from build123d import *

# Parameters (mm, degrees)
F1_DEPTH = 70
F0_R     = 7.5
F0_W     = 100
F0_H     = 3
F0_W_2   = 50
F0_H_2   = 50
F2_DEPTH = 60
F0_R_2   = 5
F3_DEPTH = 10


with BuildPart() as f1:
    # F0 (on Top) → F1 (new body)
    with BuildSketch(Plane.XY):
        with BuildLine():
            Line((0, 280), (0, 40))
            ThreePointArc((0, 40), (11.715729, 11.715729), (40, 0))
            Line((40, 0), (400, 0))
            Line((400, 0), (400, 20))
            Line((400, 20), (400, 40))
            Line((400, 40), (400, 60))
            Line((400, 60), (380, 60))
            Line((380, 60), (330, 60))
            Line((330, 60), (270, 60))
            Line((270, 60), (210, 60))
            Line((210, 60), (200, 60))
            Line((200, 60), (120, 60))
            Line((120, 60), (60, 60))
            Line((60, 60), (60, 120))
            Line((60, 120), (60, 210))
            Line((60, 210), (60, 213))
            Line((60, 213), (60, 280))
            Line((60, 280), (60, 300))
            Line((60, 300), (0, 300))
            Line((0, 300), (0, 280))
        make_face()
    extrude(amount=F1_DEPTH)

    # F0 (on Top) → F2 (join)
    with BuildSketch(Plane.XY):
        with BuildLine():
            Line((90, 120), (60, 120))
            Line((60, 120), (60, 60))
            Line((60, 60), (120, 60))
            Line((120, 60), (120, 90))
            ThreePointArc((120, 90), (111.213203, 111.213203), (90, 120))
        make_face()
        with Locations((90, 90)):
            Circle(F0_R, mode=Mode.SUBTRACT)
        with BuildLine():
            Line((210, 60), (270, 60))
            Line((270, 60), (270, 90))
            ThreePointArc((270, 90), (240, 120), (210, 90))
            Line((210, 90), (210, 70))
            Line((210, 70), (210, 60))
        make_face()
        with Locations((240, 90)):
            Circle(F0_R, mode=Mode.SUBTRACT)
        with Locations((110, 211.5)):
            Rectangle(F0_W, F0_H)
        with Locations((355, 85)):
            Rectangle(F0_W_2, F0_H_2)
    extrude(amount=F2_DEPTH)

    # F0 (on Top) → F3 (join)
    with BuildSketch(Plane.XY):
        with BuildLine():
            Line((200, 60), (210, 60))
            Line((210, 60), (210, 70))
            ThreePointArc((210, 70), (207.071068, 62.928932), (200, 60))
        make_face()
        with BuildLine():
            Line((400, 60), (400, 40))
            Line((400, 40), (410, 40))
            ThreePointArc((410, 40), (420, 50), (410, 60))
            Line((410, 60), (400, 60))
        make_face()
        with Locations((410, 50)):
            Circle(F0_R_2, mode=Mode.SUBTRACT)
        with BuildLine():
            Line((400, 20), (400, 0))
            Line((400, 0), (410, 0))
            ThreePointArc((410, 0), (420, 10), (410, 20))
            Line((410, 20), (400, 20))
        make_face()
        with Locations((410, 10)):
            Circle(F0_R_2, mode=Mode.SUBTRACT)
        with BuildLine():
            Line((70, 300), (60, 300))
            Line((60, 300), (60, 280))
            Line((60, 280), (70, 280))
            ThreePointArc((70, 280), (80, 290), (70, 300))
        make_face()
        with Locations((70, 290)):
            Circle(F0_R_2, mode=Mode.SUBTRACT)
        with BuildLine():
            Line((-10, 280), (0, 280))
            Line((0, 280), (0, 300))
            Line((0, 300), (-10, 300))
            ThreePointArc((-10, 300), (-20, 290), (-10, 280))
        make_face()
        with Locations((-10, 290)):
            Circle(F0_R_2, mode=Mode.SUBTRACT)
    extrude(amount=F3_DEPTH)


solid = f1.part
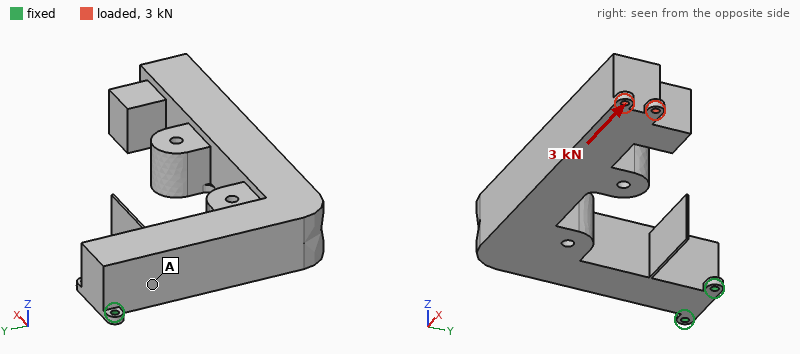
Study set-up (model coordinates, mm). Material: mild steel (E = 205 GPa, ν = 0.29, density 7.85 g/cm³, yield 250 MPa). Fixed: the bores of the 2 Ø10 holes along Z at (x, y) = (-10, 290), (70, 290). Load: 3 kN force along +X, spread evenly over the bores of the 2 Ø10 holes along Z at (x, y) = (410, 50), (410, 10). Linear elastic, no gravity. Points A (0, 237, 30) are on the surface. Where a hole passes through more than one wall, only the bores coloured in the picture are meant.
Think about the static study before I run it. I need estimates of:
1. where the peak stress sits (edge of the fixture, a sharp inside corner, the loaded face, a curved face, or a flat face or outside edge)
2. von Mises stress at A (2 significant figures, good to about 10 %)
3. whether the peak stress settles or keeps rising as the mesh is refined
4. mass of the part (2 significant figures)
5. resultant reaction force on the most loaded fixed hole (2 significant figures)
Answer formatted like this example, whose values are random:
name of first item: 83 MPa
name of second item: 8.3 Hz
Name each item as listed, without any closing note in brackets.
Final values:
where the peak stress sits: edge of the fixture
von Mises stress at A: 15 MPa
whether the peak stress settles or keeps rising as the mesh is refined: keeps rising
mass of the part: 25 kg
resultant reaction force on the most loaded fixed hole: 11 kN
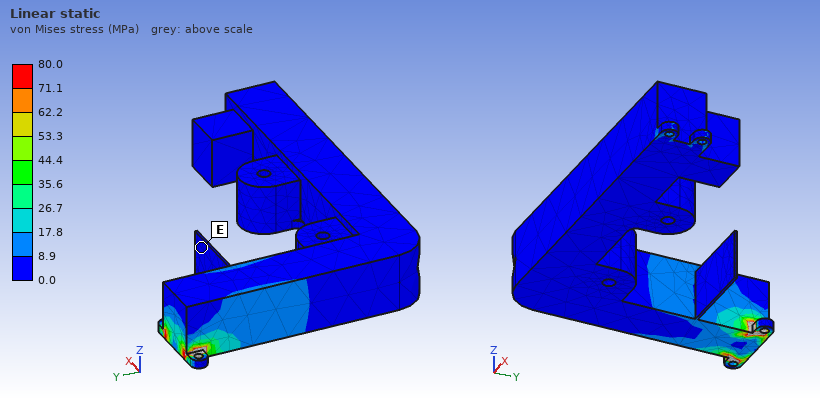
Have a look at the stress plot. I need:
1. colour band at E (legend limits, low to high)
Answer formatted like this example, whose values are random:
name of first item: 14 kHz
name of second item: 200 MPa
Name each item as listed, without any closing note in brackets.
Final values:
colour band at E: 0.0 to 8.9 MPa
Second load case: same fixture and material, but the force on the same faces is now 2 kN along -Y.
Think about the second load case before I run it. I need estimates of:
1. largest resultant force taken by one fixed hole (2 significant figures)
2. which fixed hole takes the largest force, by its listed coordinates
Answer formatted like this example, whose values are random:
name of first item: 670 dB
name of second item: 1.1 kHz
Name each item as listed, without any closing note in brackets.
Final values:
largest resultant force taken by one fixed hole: 12 kN
which fixed hole takes the largest force, by its listed coordinates: (70, 290)
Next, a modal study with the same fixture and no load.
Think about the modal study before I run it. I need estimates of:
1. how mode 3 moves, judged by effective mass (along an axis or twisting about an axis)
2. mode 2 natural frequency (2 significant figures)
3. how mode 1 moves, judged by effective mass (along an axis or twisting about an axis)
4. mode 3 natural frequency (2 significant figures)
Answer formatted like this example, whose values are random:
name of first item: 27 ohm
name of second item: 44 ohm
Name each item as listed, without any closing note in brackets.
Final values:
how mode 3 moves, judged by effective mass: twisting about Y
mode 2 natural frequency: 110 Hz
how mode 1 moves, judged by effective mass: along Z
mode 3 natural frequency: 210 Hz
